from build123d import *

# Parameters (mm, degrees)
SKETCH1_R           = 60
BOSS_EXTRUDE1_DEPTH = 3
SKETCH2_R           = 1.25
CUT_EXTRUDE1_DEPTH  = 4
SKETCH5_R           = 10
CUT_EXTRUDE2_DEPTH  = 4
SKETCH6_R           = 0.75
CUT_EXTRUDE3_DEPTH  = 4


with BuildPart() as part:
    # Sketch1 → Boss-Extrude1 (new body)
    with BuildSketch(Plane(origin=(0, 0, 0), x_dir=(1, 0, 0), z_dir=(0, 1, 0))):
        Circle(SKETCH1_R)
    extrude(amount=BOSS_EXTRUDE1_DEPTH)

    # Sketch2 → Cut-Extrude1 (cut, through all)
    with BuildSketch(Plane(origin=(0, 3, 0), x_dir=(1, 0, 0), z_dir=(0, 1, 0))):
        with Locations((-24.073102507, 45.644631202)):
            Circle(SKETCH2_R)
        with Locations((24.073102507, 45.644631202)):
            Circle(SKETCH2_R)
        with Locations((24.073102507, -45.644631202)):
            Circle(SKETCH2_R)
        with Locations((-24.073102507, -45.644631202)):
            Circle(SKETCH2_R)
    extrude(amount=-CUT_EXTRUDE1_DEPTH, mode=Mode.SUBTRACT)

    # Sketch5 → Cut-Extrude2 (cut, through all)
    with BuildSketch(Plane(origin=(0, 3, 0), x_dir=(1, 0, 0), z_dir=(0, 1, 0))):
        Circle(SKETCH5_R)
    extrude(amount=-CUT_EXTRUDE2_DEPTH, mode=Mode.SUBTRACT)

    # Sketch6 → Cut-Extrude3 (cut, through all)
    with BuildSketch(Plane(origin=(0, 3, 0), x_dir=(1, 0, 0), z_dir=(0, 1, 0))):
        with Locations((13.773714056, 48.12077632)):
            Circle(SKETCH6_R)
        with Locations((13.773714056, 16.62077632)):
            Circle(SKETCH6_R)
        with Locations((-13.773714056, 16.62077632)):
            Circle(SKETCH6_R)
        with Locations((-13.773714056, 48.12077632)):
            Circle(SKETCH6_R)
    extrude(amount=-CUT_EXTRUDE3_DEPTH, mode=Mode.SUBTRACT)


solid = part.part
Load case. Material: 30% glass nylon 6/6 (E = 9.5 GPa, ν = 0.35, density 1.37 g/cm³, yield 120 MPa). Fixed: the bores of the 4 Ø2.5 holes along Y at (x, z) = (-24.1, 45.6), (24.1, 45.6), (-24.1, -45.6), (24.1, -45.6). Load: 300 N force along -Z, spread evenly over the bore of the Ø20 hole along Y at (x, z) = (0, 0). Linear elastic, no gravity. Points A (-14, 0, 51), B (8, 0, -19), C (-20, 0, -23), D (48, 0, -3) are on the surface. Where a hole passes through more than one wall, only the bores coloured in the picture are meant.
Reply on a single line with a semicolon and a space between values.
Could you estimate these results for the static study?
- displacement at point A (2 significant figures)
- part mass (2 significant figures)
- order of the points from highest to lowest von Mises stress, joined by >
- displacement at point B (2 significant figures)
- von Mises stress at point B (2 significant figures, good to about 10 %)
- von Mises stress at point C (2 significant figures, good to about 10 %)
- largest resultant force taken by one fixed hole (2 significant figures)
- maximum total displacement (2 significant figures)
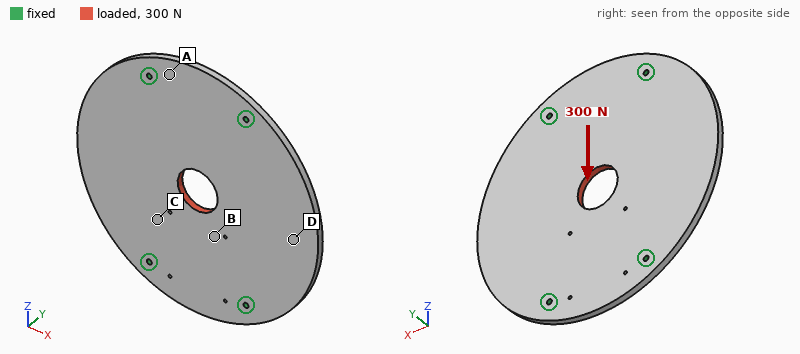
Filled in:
2.3 µm; 45 g; B > C > A > D; 4.8 µm; 1.2 MPa; 0.87 MPa; 76 N; 6.6 µm
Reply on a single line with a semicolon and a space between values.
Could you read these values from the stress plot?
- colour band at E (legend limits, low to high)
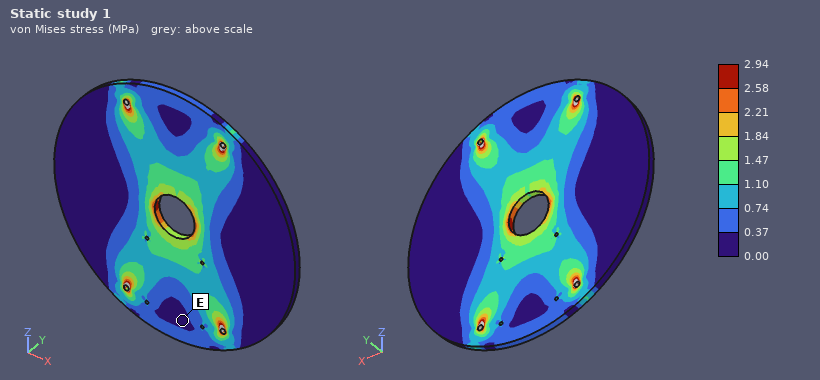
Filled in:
0.00 to 0.37 MPa
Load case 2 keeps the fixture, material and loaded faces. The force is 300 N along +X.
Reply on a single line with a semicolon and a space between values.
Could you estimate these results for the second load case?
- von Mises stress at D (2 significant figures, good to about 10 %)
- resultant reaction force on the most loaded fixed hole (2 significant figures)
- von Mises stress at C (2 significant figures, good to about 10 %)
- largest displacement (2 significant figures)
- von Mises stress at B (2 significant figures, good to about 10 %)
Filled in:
0.69 MPa; 77 N; 0.92 MPa; 9.8 µm; 1.2 MPa
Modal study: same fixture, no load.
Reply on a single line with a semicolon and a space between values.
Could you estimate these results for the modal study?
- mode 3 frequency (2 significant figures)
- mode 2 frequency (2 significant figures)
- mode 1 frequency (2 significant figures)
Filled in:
1100 Hz; 640 Hz; 640 Hz
